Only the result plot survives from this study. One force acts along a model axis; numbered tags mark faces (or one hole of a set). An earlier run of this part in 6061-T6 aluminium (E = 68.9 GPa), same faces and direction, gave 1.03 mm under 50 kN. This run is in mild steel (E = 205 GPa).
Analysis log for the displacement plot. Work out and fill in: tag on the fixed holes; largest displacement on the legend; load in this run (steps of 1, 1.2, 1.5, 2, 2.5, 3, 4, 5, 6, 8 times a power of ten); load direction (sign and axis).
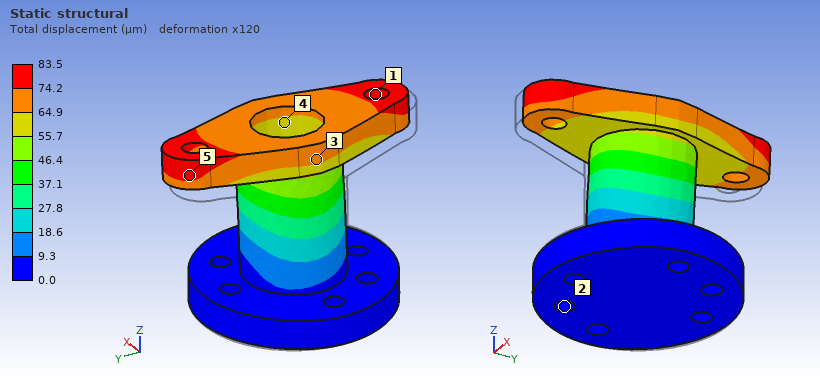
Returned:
2
83.5 µm
12 kN
+X
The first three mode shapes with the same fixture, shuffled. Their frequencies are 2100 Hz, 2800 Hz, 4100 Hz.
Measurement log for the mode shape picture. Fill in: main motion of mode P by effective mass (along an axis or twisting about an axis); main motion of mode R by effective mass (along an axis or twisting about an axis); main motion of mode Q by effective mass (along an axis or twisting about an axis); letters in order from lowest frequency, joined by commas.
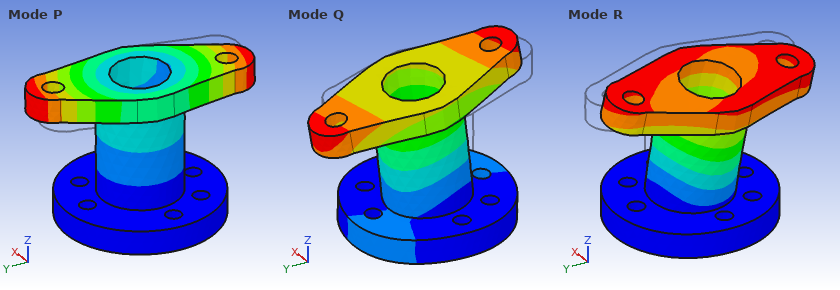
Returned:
twisting about Z
along X
along Y
Q, R, P
